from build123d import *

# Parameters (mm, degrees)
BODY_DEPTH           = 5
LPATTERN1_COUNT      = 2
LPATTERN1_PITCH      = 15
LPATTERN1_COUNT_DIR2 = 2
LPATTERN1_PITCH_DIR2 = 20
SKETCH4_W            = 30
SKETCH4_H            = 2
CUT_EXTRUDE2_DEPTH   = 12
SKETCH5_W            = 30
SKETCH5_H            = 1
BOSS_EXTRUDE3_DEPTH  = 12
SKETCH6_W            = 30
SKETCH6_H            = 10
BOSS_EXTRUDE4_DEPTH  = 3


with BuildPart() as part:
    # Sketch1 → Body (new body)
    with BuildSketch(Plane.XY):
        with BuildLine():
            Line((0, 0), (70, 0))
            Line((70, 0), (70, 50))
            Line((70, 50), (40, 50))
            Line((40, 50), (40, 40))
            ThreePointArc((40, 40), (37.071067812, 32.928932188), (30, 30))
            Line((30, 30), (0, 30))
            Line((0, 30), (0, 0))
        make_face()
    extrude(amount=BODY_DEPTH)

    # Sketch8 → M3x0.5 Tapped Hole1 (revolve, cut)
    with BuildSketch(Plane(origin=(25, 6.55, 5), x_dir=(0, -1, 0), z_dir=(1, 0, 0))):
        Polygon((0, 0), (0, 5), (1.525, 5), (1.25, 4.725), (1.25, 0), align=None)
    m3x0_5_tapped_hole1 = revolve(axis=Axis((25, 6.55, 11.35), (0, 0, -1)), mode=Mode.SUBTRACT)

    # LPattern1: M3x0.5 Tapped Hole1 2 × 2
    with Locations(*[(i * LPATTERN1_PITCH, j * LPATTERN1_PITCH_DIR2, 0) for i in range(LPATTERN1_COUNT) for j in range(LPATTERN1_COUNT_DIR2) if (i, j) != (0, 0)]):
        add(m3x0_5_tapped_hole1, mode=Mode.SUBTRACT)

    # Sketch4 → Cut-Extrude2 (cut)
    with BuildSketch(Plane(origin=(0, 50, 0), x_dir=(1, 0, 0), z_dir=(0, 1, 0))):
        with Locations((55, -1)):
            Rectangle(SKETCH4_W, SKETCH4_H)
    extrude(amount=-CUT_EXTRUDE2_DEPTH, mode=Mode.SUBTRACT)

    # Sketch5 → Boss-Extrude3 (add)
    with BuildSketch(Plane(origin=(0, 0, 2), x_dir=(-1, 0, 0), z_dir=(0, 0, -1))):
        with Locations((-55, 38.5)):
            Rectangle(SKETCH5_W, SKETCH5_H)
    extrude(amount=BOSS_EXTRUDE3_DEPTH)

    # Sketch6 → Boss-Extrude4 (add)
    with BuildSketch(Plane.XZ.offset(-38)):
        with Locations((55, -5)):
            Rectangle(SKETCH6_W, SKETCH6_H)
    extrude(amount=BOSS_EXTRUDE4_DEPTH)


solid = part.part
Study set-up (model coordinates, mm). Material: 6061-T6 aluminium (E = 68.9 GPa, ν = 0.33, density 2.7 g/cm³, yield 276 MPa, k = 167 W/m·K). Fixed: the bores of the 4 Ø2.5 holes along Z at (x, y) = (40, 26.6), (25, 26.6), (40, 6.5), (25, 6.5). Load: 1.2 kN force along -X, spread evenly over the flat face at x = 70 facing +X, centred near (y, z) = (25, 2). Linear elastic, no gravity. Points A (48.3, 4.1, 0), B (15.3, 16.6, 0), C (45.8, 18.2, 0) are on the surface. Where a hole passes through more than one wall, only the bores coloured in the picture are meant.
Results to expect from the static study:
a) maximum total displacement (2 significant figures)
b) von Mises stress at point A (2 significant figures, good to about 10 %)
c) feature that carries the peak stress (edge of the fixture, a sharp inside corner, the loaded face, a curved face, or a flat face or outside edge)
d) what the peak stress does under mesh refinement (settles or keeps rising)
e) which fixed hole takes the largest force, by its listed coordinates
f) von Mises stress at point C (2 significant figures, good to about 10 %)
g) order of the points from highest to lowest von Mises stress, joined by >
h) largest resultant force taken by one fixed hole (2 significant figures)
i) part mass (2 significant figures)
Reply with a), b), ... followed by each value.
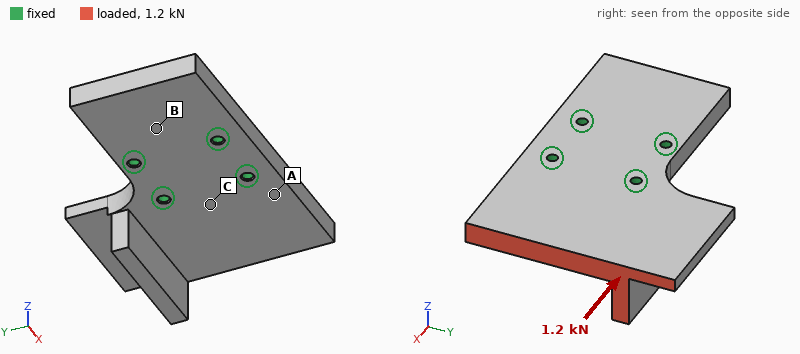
a) 25 µm
b) 5.2 MPa
c) edge of the fixture
d) keeps rising
e) (40, 26.6)
f) 8.9 MPa
g) C > A > B
h) 840 N
i) 38 g
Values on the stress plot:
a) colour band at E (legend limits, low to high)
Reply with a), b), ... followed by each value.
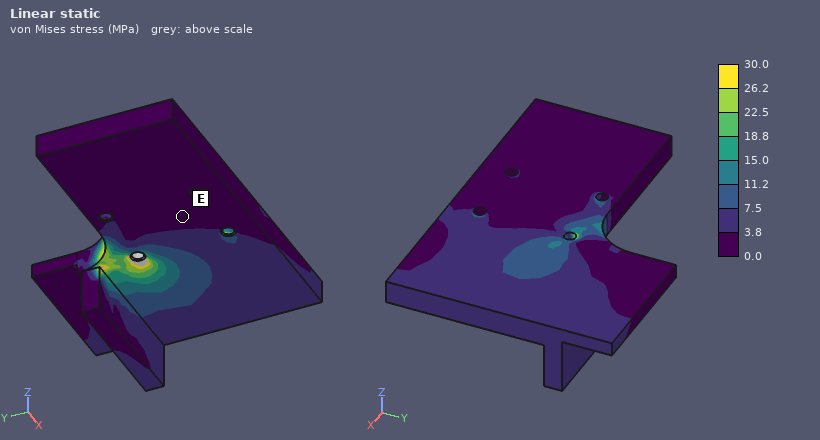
a) 0.0 to 3.8 MPa
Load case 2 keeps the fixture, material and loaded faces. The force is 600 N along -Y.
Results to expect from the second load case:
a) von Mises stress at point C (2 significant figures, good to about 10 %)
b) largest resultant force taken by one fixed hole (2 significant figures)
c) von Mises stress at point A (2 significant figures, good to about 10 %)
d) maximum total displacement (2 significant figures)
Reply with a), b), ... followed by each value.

a) 12 MPa
b) 740 N
c) 9.5 MPa
d) 27 µm
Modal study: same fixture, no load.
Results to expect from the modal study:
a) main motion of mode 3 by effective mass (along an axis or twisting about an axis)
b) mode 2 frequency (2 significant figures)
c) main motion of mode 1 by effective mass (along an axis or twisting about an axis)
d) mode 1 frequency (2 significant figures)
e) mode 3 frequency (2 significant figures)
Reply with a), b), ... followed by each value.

a) along Z
b) 5400 Hz
c) along Z
d) 3200 Hz
e) 5900 Hz
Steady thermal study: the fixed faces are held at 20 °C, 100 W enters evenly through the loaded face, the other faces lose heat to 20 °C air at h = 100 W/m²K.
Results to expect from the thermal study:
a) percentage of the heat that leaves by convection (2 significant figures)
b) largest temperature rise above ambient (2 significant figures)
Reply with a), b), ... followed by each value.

a) 19 %
b) 80 K
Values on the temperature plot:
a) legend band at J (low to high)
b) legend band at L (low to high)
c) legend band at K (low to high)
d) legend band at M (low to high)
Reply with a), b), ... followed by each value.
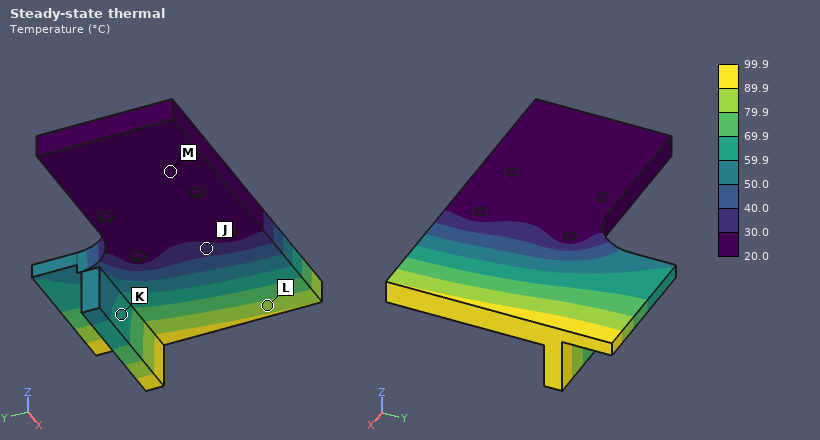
a) 30.0 to 40.0 °C
b) 79.9 to 89.9 °C
c) 59.9 to 69.9 °C
d) 20.0 to 30.0 °C
